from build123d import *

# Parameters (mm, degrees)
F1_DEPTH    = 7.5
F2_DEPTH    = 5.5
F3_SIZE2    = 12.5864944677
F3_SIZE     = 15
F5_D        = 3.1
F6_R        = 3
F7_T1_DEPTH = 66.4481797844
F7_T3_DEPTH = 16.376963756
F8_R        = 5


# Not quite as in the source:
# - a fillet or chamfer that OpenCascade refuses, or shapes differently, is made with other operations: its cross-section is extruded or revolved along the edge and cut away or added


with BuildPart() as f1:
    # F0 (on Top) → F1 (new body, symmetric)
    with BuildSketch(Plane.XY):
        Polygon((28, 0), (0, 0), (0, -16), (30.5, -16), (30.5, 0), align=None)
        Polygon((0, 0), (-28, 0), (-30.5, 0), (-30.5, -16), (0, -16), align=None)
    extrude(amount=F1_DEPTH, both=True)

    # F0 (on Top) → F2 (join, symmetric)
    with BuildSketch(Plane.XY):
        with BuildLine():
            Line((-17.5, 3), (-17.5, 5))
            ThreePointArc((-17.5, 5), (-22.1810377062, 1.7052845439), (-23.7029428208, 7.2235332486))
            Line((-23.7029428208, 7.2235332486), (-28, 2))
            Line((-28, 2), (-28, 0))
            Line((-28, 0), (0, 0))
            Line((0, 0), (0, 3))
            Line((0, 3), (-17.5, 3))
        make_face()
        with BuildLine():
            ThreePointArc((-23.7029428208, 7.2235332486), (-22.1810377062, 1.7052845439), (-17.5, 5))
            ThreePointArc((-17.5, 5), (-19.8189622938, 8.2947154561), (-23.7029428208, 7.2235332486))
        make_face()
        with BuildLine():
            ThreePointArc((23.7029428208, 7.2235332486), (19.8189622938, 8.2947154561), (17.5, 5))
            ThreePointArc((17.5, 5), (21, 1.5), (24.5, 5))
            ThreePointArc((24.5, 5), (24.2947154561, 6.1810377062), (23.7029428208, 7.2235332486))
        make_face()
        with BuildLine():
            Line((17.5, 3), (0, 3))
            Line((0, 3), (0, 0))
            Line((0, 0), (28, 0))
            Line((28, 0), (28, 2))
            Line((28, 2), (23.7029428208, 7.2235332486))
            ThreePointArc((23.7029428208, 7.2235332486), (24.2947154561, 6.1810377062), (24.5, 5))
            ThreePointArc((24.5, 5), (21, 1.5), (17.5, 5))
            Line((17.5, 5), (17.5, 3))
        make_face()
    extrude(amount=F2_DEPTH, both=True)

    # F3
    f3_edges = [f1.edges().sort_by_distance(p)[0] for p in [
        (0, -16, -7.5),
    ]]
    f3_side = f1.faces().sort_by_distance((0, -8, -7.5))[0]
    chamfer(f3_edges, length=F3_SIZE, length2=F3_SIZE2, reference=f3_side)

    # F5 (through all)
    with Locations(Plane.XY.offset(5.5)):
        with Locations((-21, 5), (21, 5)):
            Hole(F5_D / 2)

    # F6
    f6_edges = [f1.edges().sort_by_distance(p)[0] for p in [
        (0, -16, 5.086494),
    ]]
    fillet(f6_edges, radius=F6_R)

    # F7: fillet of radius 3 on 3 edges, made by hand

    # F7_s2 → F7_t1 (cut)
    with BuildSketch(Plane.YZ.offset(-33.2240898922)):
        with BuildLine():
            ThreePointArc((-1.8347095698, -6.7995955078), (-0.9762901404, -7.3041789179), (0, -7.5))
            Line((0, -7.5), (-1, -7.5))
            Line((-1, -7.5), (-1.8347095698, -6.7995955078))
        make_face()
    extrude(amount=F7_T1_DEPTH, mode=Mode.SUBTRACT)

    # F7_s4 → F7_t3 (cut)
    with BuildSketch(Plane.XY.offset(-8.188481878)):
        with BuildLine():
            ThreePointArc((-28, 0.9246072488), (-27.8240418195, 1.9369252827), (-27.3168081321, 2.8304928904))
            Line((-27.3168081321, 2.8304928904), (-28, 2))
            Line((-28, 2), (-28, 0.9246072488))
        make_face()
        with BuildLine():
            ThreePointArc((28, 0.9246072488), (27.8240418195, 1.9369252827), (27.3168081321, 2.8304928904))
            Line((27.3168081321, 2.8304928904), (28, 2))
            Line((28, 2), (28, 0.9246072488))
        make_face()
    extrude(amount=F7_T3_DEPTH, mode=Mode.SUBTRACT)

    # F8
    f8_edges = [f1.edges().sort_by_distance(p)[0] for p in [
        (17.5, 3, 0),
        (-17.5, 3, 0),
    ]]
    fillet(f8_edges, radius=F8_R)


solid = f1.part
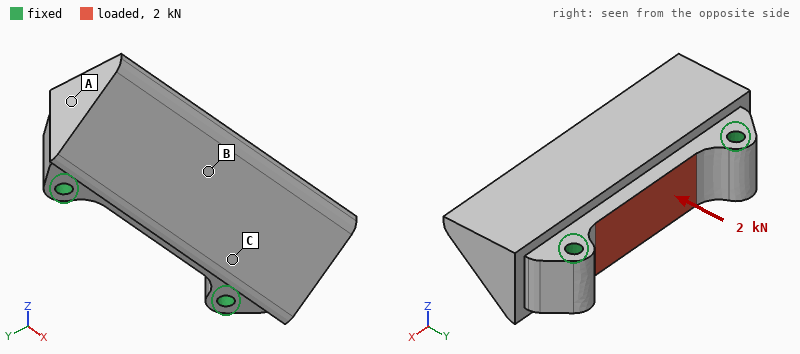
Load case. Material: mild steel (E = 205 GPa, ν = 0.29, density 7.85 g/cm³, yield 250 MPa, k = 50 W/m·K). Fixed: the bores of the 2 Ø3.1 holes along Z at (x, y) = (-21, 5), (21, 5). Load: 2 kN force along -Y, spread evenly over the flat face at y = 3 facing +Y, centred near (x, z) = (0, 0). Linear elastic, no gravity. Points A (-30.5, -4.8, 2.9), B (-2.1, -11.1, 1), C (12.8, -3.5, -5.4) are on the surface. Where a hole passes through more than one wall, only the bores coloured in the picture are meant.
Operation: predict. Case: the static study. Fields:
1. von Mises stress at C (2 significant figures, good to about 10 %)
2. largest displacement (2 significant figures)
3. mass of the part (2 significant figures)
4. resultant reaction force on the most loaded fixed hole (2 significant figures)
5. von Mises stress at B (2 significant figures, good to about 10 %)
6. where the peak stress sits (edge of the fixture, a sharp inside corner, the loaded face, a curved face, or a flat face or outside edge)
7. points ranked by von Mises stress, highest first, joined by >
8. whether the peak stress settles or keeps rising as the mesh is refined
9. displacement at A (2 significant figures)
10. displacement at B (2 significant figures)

12 MPa
3.4 µm
90 g
1.2 kN
18 MPa
edge of the fixture
B > C > A
keeps rising
0.62 µm
2.3 µm
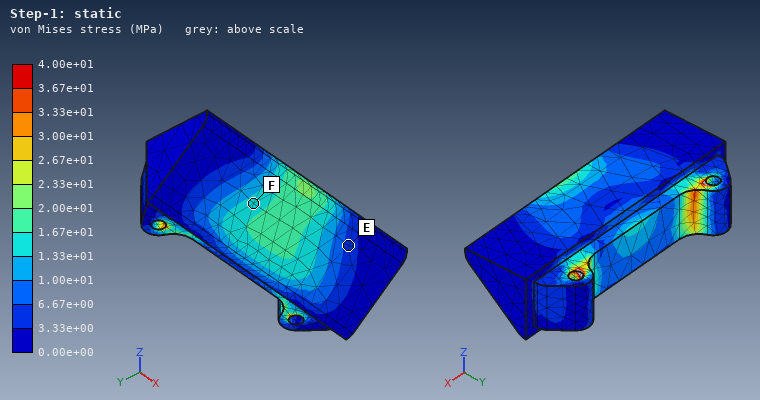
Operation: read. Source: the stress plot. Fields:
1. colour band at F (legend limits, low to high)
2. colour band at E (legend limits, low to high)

1.33e+01 to 1.67e+01 MPa
3.33e+00 to 6.67e+00 MPa
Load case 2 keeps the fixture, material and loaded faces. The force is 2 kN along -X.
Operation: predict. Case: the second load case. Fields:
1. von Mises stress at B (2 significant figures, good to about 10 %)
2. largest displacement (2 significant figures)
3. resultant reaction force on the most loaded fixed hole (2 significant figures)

4.6 MPa
1.8 µm
1.0 kN
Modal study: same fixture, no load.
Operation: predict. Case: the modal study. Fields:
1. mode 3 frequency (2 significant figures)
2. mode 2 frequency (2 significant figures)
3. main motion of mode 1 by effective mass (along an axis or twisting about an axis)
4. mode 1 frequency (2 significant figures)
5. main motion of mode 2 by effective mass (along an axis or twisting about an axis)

21 kHz
19 kHz
along Z
12 kHz
twisting about Y
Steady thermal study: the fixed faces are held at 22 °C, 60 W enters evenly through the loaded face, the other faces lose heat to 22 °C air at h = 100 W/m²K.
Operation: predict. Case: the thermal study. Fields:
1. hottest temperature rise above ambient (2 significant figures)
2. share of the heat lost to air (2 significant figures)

79 K
19 %
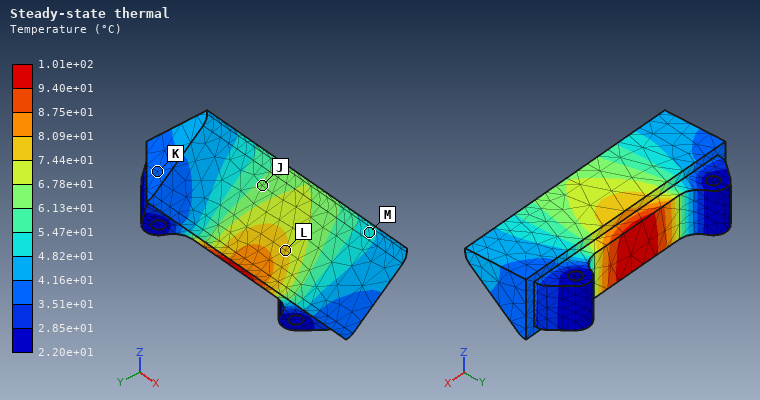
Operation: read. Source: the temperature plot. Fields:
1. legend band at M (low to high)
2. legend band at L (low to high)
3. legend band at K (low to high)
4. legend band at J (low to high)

4.82e+01 to 5.47e+01 °C
7.44e+01 to 8.09e+01 °C
3.51e+01 to 4.16e+01 °C
6.13e+01 to 6.78e+01 °C
